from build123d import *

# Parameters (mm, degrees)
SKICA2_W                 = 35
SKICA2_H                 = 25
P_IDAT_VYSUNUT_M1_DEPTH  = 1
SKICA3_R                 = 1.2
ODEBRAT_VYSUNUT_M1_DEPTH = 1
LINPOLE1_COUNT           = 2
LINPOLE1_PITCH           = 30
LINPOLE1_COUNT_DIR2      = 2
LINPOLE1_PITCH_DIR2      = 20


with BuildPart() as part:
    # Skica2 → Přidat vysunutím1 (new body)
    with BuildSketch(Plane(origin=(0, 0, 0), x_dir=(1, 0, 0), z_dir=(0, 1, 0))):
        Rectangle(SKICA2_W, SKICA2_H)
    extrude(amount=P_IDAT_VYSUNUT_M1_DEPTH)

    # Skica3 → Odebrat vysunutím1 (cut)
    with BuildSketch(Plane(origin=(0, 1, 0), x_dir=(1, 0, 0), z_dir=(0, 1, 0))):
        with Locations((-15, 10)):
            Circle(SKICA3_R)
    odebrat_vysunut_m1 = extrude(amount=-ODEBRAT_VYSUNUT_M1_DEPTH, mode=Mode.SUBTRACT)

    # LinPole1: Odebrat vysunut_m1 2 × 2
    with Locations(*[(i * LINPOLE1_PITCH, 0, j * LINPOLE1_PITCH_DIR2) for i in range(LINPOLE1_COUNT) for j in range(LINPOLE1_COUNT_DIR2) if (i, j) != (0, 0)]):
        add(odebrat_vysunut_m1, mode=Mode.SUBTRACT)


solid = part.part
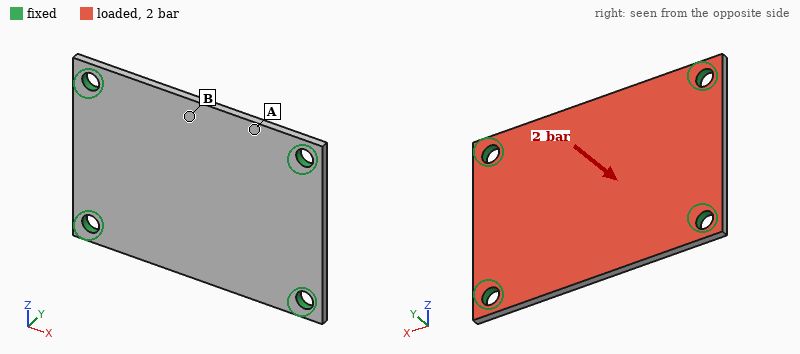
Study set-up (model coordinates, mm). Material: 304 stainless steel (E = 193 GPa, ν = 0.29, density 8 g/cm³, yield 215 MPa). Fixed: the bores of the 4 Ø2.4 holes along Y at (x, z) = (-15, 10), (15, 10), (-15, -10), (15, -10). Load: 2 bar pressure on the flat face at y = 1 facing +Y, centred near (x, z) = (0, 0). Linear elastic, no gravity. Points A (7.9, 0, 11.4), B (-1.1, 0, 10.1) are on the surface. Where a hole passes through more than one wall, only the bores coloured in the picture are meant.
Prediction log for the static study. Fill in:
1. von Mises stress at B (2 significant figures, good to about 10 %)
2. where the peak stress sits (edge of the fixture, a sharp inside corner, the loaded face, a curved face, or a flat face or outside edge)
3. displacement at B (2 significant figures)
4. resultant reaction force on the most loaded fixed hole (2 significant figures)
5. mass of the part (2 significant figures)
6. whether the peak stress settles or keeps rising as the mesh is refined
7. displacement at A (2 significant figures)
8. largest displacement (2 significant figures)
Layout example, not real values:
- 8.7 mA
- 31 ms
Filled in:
- 48 MPa
- edge of the fixture
- 28 µm
- 43 N
- 6.9 g
- keeps rising
- 13 µm
- 32 µm
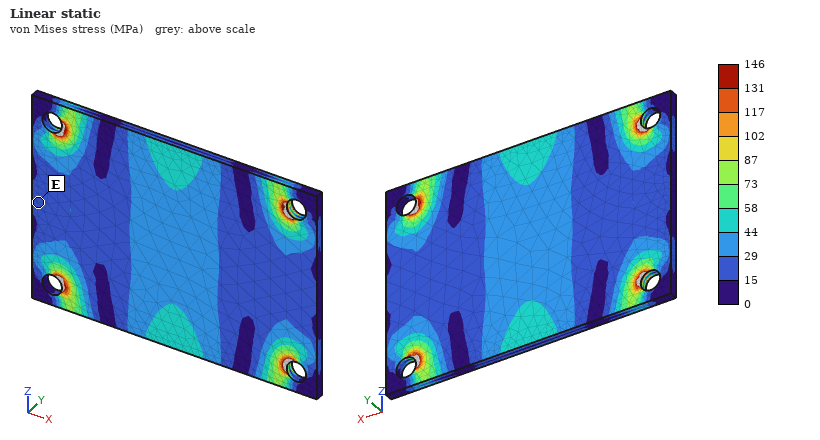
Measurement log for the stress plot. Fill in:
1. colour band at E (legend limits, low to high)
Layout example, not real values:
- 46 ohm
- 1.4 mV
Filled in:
- 15 to 29 MPa
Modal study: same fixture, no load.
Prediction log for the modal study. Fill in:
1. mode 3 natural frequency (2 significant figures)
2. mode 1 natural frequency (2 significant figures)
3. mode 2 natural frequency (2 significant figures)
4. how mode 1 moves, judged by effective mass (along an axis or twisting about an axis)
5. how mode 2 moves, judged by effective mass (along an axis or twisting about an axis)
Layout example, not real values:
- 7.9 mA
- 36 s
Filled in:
- 12 kHz
- 5200 Hz
- 7700 Hz
- along Y
- twisting about X
